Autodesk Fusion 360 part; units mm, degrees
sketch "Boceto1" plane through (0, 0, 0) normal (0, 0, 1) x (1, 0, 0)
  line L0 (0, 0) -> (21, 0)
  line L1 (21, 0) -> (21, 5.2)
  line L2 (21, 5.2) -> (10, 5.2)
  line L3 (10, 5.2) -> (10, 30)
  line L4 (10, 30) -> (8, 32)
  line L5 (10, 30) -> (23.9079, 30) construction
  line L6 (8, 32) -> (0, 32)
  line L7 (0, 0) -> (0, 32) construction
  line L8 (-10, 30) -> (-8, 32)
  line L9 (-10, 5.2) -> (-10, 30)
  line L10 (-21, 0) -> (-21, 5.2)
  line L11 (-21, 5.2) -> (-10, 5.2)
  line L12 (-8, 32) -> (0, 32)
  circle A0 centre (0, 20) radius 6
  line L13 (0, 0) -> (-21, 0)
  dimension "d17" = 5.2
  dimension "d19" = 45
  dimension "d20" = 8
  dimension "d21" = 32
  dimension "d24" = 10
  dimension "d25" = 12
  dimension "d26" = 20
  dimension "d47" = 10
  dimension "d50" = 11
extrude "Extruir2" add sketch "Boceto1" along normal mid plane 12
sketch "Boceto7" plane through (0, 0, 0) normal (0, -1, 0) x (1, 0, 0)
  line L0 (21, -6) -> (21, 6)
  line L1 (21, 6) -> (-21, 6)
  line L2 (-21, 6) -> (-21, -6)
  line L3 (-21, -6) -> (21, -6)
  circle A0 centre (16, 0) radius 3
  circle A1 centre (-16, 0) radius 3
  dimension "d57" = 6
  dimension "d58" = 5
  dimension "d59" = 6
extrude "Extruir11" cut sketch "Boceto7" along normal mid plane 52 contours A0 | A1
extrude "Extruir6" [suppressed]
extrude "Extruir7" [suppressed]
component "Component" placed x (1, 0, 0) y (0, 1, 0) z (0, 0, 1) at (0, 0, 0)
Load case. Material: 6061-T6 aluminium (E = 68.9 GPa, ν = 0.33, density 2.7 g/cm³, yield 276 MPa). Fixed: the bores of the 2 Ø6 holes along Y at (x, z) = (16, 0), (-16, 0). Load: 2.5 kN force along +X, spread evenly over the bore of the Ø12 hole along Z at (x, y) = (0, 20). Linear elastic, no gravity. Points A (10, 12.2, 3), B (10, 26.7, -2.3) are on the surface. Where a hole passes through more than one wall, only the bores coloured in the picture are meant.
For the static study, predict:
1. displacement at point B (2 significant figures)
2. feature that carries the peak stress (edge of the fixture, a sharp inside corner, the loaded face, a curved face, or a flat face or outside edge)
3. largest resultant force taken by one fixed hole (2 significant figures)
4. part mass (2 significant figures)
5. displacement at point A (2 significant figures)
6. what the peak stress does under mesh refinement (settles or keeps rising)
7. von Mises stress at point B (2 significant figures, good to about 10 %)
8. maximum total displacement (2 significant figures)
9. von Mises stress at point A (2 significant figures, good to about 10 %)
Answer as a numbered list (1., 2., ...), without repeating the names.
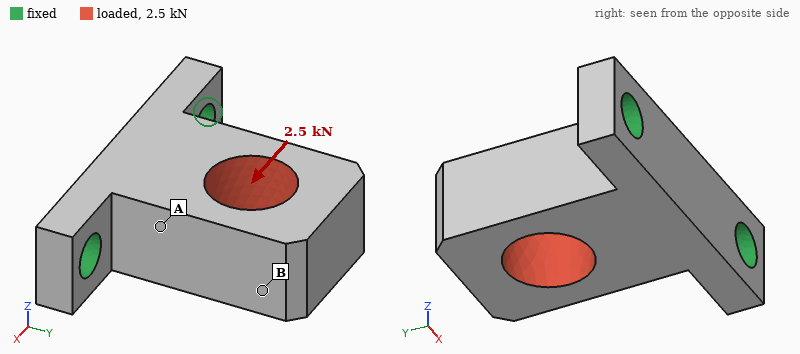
1. 59 µm
2. edge of the fixture
3. 2.2 kN
4. 20 g
5. 21 µm
6. keeps rising
7. 21 MPa
8. 67 µm
9. 51 MPa
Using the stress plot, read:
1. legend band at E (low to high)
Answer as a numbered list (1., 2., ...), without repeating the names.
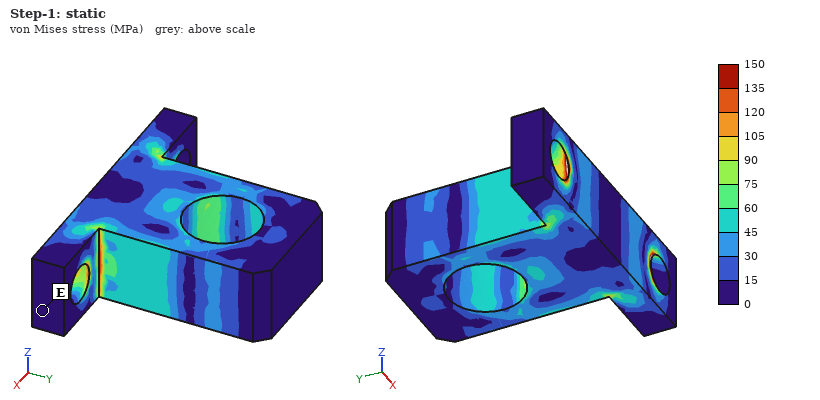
1. 0 to 15 MPa
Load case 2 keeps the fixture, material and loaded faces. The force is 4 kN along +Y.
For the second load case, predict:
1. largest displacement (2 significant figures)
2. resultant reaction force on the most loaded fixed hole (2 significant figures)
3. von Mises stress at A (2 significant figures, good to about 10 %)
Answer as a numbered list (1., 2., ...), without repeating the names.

1. 23 µm
2. 2.1 kN
3. 31 MPa
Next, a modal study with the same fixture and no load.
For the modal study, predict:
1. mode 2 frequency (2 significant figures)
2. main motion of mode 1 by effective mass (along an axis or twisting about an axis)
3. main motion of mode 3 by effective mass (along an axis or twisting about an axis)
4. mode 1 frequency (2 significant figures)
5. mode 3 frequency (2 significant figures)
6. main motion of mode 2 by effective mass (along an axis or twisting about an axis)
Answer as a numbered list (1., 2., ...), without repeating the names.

1. 10 kHz
2. along Z
3. twisting about Y
4. 4700 Hz
5. 18 kHz
6. along X
